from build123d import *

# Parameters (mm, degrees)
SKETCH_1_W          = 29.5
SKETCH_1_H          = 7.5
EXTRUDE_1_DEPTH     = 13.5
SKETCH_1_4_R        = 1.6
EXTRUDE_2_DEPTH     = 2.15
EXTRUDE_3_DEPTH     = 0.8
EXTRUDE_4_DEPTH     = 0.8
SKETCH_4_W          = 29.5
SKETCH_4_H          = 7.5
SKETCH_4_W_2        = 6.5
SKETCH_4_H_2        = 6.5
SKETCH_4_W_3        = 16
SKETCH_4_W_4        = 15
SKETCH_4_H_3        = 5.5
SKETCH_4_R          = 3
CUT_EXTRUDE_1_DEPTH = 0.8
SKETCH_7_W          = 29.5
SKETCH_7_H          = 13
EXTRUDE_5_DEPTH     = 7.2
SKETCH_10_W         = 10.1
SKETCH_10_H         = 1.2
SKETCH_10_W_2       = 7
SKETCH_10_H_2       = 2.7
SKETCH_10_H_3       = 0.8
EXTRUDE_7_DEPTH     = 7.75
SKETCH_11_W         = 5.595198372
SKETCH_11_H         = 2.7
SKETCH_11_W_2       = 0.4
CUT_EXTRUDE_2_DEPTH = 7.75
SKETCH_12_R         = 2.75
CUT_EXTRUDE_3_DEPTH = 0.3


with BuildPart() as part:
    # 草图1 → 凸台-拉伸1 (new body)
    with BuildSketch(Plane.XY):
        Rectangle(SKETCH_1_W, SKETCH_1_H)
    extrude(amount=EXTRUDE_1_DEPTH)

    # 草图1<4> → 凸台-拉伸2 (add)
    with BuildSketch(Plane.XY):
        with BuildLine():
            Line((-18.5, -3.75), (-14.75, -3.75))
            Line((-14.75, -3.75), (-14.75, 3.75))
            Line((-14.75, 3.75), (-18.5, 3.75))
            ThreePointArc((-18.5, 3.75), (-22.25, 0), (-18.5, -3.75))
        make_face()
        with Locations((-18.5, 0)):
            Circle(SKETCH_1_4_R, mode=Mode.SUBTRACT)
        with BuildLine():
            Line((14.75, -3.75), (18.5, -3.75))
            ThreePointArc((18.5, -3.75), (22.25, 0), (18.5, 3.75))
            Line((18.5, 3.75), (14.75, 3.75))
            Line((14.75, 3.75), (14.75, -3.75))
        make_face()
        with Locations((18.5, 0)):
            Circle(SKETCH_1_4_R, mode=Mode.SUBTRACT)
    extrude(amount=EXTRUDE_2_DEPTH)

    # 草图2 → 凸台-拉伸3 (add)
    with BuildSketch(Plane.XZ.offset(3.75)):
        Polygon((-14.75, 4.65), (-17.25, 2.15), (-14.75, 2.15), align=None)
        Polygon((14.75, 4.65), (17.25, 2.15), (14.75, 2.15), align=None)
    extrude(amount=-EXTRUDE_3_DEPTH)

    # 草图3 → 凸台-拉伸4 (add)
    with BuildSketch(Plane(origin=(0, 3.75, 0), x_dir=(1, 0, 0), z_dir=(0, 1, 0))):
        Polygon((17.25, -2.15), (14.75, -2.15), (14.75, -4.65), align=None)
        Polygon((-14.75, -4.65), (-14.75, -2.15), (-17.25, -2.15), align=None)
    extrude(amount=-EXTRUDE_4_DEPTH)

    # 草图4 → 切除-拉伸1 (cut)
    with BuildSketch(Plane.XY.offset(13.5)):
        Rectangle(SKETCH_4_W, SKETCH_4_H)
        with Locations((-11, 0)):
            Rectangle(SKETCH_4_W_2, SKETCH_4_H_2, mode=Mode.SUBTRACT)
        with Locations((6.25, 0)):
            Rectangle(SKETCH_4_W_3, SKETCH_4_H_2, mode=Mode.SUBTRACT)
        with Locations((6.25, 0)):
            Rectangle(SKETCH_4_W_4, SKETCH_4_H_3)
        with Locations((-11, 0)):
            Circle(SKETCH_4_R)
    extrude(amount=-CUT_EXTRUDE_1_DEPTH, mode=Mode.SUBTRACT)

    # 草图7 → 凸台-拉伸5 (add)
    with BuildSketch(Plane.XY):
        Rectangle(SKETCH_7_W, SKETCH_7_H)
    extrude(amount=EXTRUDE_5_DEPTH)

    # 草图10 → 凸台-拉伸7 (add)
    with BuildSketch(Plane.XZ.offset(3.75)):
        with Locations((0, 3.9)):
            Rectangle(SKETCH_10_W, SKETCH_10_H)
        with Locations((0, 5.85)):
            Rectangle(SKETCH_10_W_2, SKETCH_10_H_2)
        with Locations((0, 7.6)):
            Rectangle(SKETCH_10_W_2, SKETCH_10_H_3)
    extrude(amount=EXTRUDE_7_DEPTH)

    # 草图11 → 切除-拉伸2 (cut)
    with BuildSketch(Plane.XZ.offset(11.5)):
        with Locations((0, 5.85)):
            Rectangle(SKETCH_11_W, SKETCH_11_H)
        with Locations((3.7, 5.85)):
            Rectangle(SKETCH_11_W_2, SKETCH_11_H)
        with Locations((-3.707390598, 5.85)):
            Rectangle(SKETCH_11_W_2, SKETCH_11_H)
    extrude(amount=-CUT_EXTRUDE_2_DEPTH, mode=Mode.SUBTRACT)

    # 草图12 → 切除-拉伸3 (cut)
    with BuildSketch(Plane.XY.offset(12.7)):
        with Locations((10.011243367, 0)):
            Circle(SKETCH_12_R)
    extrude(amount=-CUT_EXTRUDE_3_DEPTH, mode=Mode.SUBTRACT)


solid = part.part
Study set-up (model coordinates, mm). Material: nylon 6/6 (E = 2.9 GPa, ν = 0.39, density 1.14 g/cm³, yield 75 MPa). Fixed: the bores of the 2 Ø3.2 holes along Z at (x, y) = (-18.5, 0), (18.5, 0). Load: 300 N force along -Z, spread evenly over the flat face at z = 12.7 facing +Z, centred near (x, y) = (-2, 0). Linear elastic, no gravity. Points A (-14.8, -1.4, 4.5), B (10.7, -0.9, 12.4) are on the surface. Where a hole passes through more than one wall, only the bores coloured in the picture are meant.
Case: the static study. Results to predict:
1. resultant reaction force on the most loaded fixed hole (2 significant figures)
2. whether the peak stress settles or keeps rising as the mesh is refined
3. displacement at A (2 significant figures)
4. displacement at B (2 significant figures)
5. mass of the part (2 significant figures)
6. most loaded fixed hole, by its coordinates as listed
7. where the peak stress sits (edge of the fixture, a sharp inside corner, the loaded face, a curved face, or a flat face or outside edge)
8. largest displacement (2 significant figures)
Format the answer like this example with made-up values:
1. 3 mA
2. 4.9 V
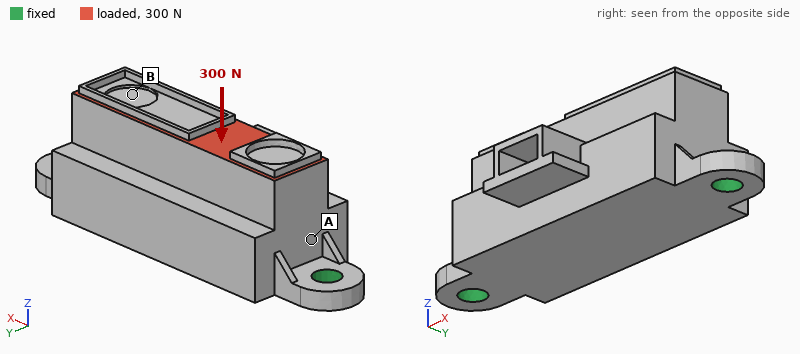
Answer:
1. 200 N
2. keeps rising
3. 72 µm
4. 68 µm
5. 4.9 g
6. (-18.5, 0)
7. edge of the fixture
8. 97 µm
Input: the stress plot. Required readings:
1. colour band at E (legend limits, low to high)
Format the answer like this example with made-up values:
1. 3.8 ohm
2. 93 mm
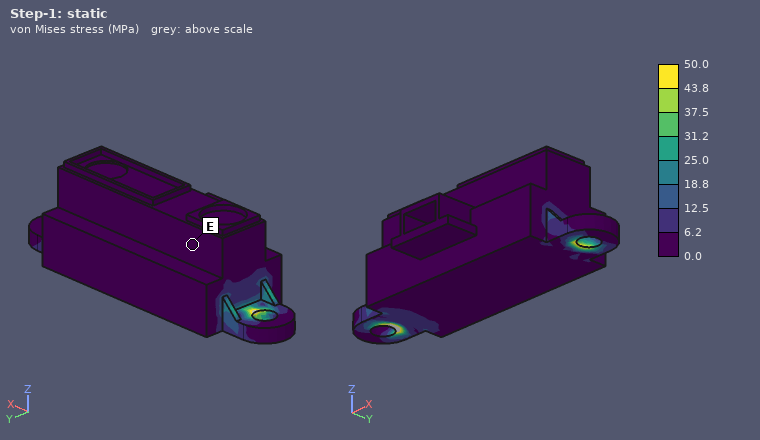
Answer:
1. 0.0 to 6.2 MPa
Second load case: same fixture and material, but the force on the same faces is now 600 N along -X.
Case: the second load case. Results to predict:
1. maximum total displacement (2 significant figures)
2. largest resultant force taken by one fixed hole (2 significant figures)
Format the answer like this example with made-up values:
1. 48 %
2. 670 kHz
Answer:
1. 0.16 mm
2. 380 N
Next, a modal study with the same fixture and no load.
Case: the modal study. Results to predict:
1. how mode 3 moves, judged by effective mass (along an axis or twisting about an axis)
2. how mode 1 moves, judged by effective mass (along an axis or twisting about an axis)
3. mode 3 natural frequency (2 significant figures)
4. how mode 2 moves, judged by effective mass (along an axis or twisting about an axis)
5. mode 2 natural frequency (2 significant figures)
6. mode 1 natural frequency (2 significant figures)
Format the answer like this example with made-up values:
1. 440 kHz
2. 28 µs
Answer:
1. along Y
2. along Y
3. 6300 Hz
4. along Z
5. 4500 Hz
6. 1700 Hz
